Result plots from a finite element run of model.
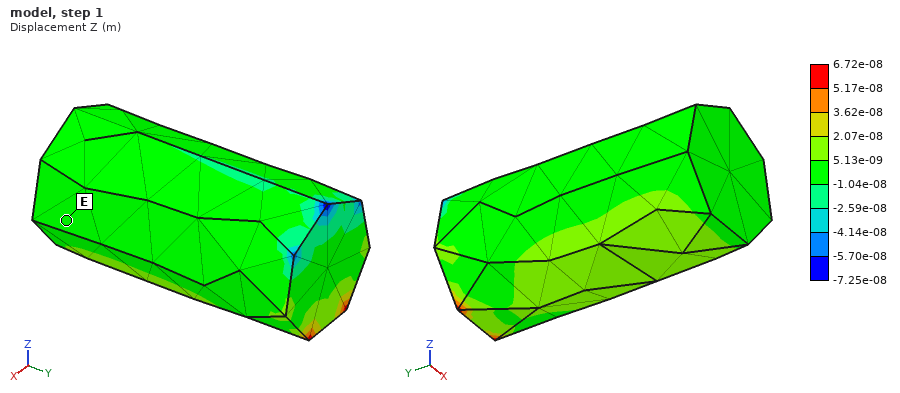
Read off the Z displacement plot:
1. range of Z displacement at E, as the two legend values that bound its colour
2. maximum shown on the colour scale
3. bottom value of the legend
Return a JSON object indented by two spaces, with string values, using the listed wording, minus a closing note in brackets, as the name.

{
  "range of Z displacement at E, as the two legend values that bound its colour": "-1.04e-08 to 5.13e-09 m",
  "maximum shown on the colour scale": "6.72e-08 m",
  "bottom value of the legend": "-7.25e-08 m"
}
